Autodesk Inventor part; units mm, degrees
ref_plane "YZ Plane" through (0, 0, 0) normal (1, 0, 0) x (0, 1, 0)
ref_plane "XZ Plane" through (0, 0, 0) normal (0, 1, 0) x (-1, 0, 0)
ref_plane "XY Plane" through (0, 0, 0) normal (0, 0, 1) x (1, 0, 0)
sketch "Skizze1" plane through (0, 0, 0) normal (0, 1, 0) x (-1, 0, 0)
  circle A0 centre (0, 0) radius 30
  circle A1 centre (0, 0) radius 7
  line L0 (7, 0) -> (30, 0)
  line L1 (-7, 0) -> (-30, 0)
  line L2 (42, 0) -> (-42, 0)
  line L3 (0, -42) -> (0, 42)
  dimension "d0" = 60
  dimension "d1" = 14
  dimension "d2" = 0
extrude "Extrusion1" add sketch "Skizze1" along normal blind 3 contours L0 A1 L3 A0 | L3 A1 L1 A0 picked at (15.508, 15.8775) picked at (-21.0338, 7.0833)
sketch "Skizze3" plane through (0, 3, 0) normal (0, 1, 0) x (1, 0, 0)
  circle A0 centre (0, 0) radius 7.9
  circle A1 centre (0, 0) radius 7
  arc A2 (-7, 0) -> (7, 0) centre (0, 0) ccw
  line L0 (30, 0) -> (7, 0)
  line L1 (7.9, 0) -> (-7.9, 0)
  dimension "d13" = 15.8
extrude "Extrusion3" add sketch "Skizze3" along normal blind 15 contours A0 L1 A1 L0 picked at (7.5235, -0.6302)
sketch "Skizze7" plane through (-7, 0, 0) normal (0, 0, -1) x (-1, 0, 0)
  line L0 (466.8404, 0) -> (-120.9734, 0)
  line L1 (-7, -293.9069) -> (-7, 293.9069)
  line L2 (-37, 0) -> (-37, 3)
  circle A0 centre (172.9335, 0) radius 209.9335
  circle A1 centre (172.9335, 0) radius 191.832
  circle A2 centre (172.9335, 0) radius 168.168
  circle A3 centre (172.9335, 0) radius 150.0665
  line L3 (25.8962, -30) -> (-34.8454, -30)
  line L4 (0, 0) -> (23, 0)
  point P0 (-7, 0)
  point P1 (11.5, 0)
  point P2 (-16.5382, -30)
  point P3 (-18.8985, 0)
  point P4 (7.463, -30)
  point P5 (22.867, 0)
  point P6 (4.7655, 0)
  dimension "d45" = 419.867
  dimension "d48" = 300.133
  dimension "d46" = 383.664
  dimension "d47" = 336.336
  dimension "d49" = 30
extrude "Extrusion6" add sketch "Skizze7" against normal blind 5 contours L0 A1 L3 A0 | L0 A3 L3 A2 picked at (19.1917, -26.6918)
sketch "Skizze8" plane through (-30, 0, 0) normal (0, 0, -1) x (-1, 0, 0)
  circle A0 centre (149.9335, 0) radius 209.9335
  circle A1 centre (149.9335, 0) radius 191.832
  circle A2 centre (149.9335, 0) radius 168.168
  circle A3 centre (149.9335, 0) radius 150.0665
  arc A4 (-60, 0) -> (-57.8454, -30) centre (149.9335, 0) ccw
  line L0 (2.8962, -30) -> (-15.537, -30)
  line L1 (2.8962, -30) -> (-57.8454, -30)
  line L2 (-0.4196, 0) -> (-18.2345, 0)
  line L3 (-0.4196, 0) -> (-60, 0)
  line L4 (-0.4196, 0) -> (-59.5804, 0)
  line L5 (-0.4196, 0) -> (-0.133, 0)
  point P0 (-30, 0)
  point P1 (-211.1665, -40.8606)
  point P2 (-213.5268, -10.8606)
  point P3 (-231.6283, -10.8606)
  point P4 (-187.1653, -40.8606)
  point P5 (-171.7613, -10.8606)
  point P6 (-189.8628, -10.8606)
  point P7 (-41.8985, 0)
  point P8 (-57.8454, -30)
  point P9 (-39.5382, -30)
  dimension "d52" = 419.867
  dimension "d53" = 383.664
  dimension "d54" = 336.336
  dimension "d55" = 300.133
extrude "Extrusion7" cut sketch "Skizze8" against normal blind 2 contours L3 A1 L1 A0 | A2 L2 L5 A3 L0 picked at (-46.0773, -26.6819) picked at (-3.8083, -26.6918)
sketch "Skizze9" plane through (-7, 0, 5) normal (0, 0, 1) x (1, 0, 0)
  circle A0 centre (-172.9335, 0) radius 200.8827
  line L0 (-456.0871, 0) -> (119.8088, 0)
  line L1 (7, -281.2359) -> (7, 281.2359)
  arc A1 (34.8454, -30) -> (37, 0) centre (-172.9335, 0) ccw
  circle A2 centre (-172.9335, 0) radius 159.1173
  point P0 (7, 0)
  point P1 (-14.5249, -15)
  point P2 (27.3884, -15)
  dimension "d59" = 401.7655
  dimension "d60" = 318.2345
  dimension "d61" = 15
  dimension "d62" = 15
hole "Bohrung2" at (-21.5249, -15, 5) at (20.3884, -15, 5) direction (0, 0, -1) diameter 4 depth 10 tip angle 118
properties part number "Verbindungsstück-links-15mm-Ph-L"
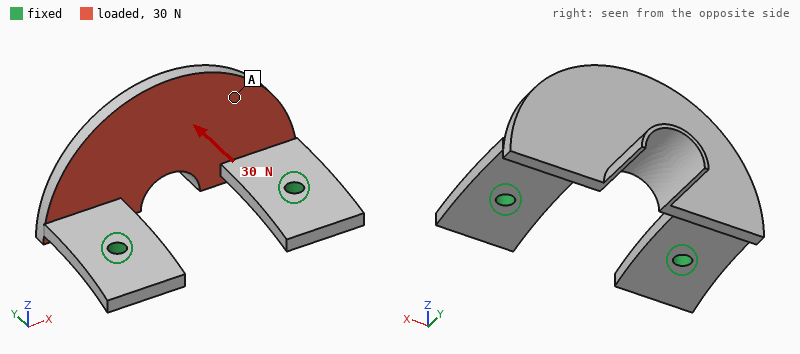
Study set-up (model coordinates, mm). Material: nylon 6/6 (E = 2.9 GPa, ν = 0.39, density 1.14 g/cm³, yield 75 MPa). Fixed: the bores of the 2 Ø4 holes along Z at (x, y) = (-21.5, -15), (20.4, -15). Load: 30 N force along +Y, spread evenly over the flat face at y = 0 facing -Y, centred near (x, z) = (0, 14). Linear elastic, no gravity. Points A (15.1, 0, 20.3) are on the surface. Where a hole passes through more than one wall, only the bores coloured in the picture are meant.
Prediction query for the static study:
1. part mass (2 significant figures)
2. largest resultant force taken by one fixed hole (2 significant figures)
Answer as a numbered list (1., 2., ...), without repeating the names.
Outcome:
1. 8.6 g
2. 16 N
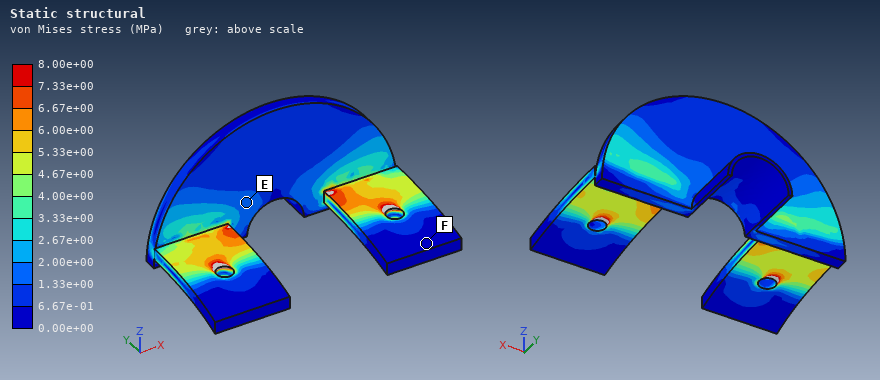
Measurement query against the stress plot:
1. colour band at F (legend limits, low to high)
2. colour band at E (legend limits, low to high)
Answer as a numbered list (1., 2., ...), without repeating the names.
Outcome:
1. 0.00e+00 to 6.67e-01 MPa
2. 1.33e+00 to 2.00e+00 MPa
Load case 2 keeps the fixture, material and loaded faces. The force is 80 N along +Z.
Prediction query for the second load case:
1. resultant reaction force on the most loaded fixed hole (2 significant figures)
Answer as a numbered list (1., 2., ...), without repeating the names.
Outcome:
1. 41 N
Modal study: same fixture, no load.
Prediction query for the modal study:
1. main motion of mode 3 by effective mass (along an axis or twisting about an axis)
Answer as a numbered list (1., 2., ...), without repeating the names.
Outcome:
1. along Z
